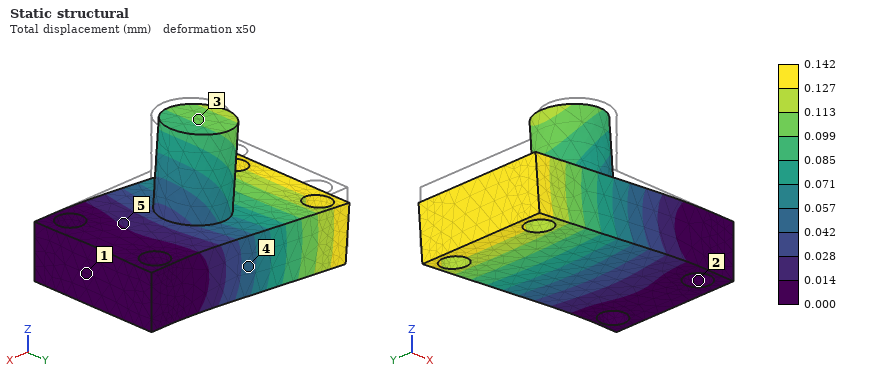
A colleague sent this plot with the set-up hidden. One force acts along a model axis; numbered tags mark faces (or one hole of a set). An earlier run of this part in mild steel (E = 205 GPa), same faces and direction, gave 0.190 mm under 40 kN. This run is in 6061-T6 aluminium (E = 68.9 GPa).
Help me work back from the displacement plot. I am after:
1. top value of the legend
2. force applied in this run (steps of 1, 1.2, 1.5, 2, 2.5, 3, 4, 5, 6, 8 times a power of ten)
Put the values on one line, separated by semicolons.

0.142 mm; 10 kN
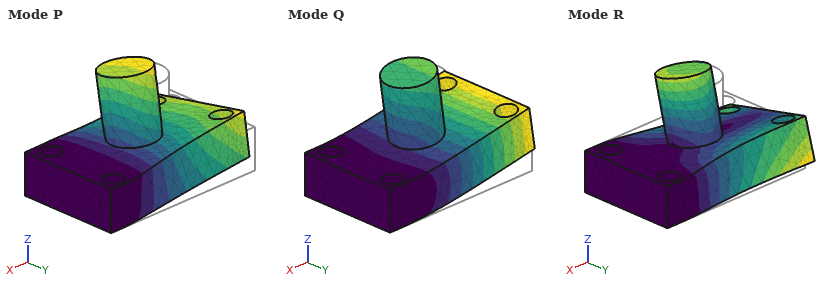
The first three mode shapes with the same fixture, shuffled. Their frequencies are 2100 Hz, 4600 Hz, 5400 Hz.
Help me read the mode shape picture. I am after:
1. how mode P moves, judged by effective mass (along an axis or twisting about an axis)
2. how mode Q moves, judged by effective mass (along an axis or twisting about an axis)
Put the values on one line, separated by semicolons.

along Y; along Z
